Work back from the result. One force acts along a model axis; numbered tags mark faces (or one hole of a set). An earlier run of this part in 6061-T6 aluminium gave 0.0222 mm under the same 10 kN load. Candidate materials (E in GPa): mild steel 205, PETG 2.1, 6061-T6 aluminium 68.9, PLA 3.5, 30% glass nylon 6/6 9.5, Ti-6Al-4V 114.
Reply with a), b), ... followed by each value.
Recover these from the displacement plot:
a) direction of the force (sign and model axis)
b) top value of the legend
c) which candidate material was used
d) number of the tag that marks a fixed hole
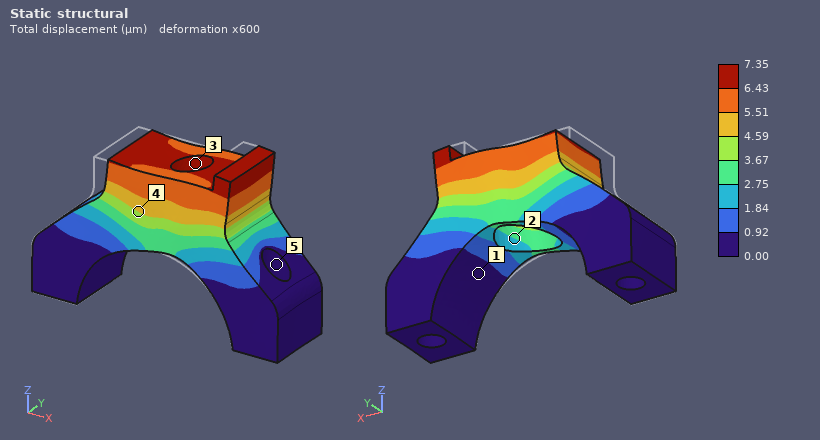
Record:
a) +X
b) 7.35 µm
c) mild steel
d) 5
